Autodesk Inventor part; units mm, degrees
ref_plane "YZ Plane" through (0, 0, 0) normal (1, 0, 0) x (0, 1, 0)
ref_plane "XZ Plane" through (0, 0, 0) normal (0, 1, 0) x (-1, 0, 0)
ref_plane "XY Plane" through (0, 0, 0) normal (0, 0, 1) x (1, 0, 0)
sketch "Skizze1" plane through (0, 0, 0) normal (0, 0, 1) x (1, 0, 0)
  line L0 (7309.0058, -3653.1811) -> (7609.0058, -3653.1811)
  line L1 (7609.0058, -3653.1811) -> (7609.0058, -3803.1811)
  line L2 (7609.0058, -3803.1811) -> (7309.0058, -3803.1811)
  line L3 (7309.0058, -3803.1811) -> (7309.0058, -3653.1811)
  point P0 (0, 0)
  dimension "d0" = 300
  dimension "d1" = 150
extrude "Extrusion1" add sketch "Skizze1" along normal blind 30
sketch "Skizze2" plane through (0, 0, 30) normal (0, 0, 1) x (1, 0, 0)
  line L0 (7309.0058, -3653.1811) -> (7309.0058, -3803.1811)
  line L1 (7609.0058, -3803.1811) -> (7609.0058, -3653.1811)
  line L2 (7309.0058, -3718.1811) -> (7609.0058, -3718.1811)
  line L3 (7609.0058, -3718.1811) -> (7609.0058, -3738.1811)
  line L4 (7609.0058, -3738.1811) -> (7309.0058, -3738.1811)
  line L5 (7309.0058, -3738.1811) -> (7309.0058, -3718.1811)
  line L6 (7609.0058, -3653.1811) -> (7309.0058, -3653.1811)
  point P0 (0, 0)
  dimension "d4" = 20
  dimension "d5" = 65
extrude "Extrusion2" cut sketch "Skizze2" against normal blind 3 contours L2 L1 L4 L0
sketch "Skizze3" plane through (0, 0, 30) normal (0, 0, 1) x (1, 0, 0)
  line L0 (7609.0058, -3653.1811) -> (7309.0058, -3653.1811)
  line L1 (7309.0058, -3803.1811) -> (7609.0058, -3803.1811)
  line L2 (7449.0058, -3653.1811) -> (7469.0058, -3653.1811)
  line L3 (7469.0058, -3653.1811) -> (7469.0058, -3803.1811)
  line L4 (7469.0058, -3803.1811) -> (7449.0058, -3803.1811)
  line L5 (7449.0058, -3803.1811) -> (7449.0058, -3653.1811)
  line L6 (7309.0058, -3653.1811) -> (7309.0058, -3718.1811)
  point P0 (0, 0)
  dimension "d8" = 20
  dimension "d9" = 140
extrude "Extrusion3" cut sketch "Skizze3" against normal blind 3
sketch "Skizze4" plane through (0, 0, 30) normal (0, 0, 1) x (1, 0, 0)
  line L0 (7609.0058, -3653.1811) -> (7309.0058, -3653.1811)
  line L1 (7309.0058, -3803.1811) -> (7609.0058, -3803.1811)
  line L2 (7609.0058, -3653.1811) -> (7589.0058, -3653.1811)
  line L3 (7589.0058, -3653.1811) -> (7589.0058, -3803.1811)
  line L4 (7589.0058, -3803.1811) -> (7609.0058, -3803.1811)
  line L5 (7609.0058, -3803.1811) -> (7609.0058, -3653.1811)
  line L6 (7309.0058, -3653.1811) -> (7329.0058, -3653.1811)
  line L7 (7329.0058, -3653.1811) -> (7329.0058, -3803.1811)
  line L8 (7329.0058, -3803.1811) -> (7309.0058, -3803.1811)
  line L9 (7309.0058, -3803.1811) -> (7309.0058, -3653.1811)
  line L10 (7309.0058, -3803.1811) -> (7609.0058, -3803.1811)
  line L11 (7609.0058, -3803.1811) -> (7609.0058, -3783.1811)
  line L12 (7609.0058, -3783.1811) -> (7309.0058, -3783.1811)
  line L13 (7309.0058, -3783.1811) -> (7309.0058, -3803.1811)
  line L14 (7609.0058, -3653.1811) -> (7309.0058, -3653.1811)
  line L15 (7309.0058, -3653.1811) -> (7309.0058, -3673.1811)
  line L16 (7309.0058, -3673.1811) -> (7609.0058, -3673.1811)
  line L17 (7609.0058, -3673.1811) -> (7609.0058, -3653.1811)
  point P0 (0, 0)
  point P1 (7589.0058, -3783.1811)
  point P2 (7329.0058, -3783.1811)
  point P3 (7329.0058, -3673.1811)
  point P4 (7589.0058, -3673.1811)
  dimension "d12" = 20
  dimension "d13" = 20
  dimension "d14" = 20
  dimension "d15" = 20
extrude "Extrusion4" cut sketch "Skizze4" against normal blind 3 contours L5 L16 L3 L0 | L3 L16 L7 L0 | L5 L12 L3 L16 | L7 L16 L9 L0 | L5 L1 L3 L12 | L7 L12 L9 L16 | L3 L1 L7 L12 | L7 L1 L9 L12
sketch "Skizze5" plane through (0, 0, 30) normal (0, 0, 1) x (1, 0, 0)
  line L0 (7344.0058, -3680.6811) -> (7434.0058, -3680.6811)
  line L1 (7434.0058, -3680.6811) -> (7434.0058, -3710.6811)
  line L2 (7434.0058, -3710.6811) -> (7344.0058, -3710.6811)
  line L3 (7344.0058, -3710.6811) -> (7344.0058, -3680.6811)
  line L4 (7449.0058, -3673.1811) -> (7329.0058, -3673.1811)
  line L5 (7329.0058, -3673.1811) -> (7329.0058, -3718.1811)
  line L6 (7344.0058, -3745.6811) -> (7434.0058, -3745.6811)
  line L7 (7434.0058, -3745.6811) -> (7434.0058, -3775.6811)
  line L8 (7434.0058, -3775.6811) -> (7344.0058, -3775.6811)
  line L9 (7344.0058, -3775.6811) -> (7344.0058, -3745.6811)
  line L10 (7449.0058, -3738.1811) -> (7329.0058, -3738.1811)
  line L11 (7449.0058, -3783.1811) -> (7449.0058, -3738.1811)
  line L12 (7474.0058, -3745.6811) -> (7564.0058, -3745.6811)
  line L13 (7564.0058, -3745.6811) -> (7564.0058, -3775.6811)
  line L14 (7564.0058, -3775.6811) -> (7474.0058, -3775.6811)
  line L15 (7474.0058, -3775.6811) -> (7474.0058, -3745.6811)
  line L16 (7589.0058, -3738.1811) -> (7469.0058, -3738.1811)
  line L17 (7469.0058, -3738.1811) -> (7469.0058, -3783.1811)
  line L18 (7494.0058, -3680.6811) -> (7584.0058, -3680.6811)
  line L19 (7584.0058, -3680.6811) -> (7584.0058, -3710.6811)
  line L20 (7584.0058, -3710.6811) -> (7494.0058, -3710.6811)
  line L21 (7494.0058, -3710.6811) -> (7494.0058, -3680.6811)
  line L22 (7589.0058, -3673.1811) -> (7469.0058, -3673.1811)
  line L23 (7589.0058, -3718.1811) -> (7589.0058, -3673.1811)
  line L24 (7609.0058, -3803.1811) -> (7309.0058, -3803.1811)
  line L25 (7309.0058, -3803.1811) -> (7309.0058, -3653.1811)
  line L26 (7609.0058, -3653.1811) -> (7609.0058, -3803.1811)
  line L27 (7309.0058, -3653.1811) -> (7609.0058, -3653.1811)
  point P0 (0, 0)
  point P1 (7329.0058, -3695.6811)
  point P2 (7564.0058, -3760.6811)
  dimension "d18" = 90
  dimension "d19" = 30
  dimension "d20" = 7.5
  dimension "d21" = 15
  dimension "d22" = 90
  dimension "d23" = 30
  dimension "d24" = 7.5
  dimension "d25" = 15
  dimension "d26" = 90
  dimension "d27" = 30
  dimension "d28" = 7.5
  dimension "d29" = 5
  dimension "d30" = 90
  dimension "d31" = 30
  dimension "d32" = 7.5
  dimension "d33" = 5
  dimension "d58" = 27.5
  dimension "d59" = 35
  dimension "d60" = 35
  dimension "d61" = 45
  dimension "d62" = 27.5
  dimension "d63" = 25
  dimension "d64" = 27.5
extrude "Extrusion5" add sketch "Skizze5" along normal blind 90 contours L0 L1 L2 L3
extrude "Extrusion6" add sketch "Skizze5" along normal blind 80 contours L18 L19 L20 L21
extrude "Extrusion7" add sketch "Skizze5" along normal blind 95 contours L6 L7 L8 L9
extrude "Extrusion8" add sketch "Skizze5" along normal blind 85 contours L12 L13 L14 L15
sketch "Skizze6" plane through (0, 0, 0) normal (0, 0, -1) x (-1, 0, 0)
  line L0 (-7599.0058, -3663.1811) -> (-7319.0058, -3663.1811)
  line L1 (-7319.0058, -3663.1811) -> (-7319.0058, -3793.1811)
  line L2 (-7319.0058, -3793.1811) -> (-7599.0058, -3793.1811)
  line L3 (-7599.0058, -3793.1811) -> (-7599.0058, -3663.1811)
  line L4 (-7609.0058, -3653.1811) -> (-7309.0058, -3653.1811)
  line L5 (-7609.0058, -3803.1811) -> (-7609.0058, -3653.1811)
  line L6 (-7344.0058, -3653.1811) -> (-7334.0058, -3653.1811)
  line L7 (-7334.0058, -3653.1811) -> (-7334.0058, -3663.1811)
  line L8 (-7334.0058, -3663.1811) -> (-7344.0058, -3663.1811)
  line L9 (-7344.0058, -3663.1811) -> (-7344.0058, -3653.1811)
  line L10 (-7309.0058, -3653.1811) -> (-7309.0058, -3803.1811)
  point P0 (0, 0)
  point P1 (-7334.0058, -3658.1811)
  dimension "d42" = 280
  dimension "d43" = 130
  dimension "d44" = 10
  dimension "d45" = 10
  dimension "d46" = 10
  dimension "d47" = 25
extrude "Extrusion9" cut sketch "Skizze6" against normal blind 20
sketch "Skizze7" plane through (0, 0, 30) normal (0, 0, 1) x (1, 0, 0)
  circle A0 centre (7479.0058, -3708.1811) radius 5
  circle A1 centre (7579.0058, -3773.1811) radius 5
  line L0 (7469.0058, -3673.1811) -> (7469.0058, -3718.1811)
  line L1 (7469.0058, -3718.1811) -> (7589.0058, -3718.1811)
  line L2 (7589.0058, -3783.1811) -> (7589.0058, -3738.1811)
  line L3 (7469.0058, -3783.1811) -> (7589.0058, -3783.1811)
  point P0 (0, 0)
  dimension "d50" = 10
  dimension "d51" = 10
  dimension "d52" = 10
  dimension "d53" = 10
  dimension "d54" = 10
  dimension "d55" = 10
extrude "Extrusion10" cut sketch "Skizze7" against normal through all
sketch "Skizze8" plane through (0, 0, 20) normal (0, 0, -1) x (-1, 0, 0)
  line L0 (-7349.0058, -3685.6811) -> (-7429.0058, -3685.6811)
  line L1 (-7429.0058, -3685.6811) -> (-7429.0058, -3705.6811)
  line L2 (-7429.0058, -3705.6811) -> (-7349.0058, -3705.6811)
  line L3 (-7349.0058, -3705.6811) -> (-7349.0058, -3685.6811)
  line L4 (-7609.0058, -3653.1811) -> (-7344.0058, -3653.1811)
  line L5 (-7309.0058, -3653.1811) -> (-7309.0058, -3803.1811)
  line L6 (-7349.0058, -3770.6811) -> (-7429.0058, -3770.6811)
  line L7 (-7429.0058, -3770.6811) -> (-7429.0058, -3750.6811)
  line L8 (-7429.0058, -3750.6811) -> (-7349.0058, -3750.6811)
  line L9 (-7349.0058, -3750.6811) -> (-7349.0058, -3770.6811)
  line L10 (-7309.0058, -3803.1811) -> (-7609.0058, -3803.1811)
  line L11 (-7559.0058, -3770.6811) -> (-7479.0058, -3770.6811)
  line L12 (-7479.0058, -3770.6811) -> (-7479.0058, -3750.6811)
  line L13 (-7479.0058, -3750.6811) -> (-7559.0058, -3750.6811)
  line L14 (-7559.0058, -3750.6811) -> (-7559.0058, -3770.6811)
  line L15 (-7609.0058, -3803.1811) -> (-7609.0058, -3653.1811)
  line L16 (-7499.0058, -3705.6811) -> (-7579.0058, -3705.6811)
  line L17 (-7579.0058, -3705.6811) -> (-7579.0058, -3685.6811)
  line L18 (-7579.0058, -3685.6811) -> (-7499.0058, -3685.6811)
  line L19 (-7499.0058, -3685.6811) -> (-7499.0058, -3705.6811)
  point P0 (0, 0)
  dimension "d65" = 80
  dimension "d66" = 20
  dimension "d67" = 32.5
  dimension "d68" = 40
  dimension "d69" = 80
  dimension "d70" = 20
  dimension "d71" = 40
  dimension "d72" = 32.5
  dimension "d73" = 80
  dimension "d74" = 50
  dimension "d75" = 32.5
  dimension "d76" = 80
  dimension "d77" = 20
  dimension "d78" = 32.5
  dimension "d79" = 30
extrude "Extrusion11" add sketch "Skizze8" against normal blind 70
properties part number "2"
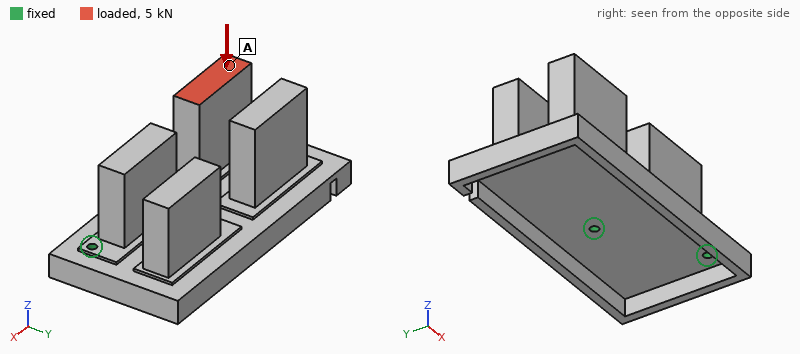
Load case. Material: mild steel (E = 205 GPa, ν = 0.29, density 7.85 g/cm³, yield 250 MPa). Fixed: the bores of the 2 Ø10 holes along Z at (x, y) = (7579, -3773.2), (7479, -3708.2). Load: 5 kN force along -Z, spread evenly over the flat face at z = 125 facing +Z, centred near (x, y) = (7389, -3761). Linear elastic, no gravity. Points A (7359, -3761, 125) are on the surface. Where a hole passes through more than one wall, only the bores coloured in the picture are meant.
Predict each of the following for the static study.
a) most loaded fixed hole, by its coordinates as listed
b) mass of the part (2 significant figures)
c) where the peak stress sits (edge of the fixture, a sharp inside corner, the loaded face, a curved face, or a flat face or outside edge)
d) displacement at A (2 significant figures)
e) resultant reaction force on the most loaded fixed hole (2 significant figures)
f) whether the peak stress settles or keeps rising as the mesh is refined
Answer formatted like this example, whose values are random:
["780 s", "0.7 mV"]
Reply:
["(7479, -3708.2)", "12 kg", "edge of the fixture", "0.85 mm", "6.9 kN", "keeps rising"]
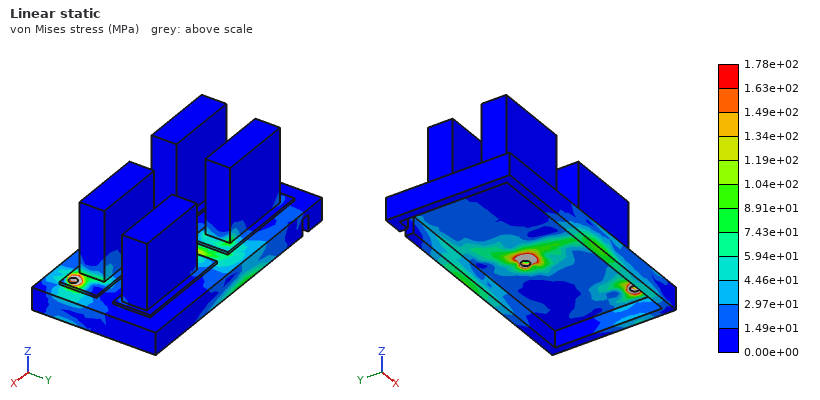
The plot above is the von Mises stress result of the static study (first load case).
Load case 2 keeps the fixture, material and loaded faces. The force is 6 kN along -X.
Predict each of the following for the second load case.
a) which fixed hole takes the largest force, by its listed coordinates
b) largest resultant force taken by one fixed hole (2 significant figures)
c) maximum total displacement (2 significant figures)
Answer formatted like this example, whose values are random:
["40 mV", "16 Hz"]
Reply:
["(7479, -3708.2)", "6.9 kN", "1.2 mm"]
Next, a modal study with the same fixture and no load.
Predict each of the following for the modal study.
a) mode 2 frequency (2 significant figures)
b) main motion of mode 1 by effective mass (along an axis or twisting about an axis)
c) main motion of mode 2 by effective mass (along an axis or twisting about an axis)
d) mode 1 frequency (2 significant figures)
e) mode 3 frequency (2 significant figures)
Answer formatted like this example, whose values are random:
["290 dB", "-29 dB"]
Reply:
["340 Hz", "along Z", "along Y", "180 Hz", "580 Hz"]
